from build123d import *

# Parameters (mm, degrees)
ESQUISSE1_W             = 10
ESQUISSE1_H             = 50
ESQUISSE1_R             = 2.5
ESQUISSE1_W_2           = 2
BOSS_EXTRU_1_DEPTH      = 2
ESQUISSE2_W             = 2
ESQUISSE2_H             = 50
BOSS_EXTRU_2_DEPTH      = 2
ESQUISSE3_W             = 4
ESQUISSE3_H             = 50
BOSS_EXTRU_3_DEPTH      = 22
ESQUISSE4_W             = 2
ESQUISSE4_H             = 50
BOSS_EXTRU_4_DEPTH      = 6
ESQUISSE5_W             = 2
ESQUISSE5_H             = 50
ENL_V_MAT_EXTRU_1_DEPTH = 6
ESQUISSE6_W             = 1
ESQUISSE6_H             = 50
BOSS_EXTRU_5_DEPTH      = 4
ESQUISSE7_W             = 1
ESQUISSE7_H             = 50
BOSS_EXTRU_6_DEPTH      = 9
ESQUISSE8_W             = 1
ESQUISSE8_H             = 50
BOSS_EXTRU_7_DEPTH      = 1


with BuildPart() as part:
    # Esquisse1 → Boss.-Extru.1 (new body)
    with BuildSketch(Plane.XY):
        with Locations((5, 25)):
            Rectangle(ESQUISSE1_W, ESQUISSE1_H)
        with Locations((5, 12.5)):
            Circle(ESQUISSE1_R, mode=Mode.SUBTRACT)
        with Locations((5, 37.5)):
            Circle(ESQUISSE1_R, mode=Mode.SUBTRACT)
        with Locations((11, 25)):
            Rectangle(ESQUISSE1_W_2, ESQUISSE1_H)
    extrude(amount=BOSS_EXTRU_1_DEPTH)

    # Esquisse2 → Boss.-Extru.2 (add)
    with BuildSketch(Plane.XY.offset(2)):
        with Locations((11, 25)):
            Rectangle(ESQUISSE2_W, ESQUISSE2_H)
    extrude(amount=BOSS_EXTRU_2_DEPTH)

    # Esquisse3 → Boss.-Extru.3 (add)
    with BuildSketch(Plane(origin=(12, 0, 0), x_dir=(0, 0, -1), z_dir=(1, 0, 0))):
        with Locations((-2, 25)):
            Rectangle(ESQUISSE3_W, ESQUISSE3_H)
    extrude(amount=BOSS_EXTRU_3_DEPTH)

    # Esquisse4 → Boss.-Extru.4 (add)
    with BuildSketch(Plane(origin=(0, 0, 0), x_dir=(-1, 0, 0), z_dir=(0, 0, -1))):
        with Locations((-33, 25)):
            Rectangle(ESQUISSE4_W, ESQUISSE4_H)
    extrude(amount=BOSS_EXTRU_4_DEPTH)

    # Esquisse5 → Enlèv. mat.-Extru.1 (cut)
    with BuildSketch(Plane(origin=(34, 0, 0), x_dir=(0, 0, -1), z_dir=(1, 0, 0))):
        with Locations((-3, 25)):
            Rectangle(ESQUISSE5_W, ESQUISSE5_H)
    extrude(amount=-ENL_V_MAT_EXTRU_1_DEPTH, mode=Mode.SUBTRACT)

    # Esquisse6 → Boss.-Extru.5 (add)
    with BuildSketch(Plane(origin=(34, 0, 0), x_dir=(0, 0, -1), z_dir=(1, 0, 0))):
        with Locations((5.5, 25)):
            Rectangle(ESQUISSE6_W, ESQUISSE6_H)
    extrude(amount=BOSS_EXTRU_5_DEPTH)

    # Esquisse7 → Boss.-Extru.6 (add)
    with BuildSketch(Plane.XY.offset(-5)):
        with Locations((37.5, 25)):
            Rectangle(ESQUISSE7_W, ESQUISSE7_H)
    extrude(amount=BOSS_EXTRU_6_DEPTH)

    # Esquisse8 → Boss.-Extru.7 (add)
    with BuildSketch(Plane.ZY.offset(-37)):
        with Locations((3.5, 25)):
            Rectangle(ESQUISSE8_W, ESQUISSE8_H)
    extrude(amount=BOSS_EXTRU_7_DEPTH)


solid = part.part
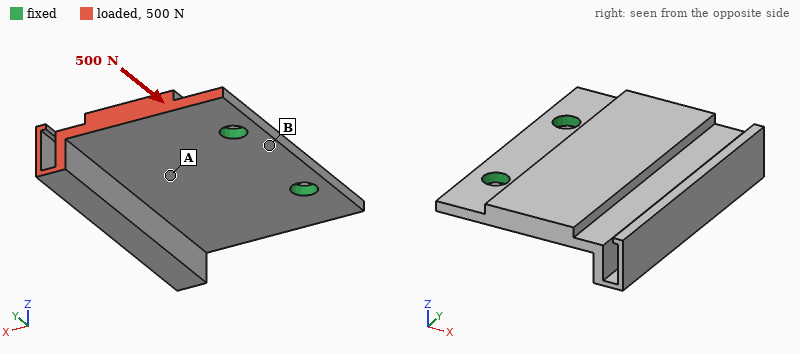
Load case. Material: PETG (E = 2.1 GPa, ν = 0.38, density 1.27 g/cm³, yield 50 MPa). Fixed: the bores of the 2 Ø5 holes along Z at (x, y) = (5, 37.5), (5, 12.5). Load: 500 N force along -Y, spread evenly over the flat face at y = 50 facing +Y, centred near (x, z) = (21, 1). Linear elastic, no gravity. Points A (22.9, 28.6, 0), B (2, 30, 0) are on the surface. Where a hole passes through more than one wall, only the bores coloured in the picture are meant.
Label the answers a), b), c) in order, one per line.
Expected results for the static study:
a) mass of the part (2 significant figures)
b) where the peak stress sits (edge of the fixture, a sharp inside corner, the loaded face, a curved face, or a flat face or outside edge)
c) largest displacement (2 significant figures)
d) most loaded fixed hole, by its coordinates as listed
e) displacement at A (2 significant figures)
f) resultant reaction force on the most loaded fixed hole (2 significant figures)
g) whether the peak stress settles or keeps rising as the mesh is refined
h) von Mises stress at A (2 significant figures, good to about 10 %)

a) 8.2 g
b) edge of the fixture
c) 0.65 mm
d) (5, 37.5)
e) 0.18 mm
f) 410 N
g) keeps rising
h) 8.8 MPa
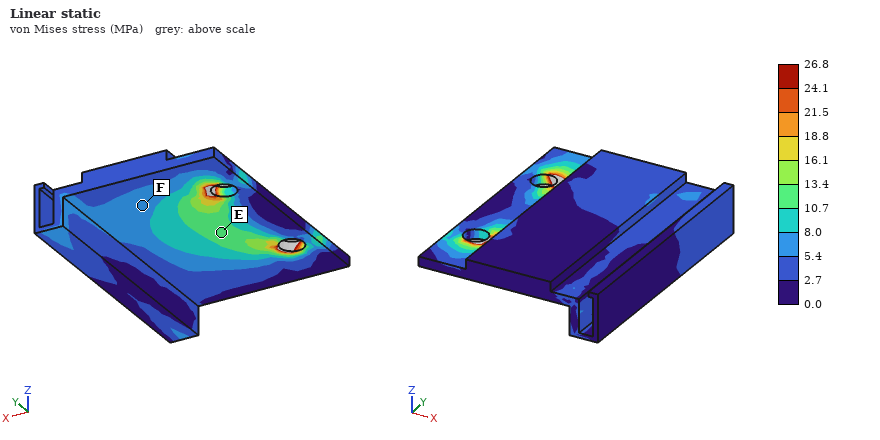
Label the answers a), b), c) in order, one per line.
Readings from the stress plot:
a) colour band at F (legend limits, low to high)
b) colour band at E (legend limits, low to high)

a) 5.4 to 8.0 MPa
b) 10.7 to 13.4 MPa
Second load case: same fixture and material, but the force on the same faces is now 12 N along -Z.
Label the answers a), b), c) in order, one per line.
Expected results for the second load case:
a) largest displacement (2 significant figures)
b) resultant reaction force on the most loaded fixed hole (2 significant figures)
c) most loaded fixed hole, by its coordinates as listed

a) 0.62 mm
b) 16 N
c) (5, 37.5)
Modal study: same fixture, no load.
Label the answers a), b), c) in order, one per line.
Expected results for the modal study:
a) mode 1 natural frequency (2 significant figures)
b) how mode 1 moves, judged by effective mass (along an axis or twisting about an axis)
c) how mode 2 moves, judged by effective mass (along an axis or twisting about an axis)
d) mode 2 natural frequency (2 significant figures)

a) 380 Hz
b) along Z
c) twisting about X
d) 820 Hz
